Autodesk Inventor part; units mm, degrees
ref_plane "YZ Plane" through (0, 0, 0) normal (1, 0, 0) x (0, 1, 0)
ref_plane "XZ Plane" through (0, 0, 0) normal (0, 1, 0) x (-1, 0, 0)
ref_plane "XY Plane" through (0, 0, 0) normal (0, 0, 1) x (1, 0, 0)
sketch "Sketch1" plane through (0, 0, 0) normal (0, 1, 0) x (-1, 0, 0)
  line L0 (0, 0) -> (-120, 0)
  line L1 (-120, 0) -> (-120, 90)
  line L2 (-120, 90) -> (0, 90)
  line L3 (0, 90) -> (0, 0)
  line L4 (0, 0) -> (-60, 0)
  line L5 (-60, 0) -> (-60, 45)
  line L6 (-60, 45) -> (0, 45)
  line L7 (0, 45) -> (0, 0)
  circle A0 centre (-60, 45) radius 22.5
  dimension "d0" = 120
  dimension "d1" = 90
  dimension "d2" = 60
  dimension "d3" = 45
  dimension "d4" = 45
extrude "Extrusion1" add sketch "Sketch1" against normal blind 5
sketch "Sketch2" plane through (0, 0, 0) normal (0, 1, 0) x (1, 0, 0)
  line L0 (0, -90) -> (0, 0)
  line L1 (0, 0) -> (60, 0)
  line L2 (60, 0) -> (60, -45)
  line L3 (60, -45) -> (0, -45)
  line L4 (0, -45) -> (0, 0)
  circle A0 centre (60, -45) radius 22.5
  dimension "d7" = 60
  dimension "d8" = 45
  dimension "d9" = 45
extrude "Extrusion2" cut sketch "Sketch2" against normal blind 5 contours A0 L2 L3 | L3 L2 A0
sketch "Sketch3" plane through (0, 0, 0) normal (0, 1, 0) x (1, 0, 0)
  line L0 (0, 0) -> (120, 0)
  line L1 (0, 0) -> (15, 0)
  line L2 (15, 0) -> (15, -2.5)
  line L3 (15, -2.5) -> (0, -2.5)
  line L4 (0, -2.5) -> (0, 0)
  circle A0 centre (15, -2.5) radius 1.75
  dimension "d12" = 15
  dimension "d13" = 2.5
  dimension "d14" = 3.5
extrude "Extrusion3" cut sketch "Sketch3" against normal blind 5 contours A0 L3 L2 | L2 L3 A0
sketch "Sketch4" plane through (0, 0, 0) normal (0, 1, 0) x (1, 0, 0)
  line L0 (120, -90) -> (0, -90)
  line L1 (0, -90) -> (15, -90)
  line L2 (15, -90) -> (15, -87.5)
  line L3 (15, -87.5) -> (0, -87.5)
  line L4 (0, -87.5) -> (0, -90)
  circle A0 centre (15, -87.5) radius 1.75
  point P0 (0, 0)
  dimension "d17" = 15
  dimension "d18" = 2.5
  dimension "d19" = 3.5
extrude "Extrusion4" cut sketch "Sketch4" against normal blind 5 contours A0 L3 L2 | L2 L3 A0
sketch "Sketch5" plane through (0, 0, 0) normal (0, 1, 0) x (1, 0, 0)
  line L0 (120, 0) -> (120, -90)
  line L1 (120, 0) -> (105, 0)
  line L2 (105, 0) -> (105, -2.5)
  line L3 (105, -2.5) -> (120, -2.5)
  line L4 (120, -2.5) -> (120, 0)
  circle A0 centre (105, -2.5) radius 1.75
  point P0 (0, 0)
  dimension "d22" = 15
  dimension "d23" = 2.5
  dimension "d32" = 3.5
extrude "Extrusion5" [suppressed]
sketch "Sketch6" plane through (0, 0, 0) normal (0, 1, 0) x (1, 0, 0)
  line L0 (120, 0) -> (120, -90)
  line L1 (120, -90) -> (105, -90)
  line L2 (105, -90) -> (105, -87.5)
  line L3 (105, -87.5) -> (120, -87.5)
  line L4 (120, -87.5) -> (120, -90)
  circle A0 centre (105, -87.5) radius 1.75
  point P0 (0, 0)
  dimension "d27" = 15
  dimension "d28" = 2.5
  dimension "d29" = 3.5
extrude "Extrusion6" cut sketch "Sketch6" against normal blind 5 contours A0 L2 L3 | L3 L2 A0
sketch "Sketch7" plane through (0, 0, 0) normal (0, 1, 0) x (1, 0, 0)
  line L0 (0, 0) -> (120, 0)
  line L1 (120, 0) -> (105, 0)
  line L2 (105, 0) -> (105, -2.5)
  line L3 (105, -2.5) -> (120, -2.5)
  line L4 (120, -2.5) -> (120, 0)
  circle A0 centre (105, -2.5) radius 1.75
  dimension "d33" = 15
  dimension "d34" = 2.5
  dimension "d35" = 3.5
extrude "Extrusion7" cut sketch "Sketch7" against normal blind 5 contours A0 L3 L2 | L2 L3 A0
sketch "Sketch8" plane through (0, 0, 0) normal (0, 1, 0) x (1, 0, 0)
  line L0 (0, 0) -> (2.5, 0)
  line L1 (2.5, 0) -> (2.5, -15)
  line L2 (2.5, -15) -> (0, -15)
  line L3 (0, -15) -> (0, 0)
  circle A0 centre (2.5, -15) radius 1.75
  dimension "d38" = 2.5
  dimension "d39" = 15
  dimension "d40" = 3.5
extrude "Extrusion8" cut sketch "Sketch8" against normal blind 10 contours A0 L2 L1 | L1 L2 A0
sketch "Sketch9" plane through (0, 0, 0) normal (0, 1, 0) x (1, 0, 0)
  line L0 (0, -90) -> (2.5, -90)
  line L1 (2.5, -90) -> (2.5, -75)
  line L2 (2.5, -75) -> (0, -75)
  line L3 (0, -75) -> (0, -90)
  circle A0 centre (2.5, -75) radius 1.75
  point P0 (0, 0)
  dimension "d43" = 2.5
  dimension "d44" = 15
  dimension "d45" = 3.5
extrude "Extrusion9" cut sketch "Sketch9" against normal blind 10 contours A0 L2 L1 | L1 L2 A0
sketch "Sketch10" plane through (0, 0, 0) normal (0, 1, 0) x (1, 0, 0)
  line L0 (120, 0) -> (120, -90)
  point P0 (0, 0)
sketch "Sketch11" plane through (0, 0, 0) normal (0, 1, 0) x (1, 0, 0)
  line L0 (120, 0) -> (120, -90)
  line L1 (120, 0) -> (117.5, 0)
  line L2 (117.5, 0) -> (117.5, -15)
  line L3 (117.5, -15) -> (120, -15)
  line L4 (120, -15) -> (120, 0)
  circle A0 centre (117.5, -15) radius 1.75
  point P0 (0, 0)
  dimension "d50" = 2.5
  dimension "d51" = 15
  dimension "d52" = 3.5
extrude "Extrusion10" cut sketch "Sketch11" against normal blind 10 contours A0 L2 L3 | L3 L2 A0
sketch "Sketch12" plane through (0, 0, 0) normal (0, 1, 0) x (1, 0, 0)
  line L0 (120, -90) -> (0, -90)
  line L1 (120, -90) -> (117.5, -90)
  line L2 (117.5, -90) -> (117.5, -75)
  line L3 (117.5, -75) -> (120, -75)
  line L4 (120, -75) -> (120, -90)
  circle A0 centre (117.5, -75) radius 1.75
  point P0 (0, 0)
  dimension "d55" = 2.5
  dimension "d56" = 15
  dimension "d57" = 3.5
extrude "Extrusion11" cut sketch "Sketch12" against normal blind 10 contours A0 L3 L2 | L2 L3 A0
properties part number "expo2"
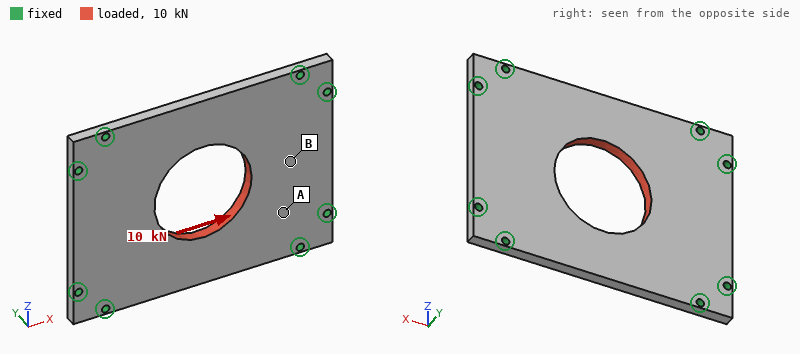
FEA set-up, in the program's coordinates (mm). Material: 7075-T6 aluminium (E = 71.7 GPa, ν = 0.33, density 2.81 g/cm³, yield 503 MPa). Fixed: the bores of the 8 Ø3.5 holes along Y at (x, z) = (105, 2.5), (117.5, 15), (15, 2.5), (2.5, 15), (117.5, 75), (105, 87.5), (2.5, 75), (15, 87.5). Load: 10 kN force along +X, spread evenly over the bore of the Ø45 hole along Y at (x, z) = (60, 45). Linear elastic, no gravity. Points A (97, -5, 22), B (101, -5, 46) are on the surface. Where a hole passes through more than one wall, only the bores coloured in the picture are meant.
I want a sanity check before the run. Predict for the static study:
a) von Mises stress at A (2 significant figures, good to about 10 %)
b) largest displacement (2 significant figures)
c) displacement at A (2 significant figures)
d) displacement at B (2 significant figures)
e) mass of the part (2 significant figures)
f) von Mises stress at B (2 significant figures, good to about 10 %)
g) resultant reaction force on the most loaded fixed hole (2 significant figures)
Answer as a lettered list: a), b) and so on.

a) 16 MPa
b) 13 µm
c) 6.6 µm
d) 11 µm
e) 130 g
f) 5.6 MPa
g) 1.6 kN
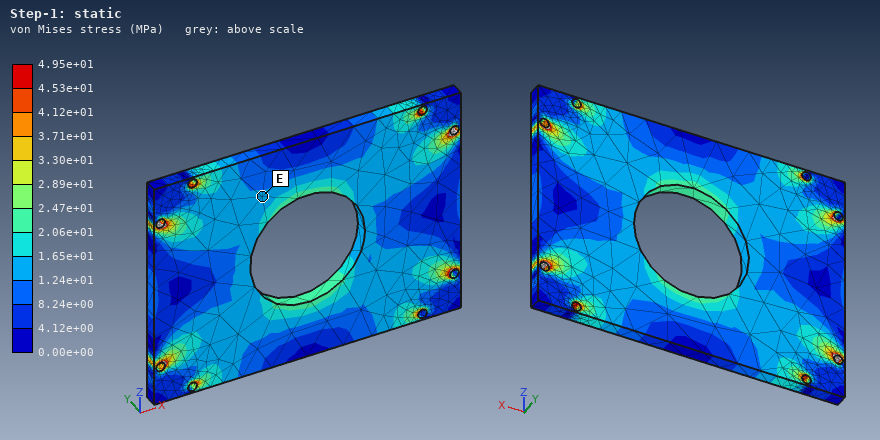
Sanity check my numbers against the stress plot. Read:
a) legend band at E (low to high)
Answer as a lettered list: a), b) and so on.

a) 1.24e+01 to 1.65e+01 MPa
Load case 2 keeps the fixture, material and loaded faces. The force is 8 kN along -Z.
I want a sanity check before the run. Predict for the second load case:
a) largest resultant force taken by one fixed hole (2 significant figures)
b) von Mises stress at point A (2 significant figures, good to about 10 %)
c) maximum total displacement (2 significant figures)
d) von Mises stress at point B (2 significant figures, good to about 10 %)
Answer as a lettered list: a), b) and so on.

a) 1.6 kN
b) 15 MPa
c) 21 µm
d) 17 MPa
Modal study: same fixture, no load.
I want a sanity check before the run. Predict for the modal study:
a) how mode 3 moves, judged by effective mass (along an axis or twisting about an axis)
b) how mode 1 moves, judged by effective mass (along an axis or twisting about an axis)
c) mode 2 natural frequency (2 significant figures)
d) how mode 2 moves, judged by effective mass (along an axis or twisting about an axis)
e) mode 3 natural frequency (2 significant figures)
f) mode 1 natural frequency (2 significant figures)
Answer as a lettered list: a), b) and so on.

a) twisting about Z
b) along Y
c) 3400 Hz
d) twisting about X
e) 4400 Hz
f) 2400 Hz
